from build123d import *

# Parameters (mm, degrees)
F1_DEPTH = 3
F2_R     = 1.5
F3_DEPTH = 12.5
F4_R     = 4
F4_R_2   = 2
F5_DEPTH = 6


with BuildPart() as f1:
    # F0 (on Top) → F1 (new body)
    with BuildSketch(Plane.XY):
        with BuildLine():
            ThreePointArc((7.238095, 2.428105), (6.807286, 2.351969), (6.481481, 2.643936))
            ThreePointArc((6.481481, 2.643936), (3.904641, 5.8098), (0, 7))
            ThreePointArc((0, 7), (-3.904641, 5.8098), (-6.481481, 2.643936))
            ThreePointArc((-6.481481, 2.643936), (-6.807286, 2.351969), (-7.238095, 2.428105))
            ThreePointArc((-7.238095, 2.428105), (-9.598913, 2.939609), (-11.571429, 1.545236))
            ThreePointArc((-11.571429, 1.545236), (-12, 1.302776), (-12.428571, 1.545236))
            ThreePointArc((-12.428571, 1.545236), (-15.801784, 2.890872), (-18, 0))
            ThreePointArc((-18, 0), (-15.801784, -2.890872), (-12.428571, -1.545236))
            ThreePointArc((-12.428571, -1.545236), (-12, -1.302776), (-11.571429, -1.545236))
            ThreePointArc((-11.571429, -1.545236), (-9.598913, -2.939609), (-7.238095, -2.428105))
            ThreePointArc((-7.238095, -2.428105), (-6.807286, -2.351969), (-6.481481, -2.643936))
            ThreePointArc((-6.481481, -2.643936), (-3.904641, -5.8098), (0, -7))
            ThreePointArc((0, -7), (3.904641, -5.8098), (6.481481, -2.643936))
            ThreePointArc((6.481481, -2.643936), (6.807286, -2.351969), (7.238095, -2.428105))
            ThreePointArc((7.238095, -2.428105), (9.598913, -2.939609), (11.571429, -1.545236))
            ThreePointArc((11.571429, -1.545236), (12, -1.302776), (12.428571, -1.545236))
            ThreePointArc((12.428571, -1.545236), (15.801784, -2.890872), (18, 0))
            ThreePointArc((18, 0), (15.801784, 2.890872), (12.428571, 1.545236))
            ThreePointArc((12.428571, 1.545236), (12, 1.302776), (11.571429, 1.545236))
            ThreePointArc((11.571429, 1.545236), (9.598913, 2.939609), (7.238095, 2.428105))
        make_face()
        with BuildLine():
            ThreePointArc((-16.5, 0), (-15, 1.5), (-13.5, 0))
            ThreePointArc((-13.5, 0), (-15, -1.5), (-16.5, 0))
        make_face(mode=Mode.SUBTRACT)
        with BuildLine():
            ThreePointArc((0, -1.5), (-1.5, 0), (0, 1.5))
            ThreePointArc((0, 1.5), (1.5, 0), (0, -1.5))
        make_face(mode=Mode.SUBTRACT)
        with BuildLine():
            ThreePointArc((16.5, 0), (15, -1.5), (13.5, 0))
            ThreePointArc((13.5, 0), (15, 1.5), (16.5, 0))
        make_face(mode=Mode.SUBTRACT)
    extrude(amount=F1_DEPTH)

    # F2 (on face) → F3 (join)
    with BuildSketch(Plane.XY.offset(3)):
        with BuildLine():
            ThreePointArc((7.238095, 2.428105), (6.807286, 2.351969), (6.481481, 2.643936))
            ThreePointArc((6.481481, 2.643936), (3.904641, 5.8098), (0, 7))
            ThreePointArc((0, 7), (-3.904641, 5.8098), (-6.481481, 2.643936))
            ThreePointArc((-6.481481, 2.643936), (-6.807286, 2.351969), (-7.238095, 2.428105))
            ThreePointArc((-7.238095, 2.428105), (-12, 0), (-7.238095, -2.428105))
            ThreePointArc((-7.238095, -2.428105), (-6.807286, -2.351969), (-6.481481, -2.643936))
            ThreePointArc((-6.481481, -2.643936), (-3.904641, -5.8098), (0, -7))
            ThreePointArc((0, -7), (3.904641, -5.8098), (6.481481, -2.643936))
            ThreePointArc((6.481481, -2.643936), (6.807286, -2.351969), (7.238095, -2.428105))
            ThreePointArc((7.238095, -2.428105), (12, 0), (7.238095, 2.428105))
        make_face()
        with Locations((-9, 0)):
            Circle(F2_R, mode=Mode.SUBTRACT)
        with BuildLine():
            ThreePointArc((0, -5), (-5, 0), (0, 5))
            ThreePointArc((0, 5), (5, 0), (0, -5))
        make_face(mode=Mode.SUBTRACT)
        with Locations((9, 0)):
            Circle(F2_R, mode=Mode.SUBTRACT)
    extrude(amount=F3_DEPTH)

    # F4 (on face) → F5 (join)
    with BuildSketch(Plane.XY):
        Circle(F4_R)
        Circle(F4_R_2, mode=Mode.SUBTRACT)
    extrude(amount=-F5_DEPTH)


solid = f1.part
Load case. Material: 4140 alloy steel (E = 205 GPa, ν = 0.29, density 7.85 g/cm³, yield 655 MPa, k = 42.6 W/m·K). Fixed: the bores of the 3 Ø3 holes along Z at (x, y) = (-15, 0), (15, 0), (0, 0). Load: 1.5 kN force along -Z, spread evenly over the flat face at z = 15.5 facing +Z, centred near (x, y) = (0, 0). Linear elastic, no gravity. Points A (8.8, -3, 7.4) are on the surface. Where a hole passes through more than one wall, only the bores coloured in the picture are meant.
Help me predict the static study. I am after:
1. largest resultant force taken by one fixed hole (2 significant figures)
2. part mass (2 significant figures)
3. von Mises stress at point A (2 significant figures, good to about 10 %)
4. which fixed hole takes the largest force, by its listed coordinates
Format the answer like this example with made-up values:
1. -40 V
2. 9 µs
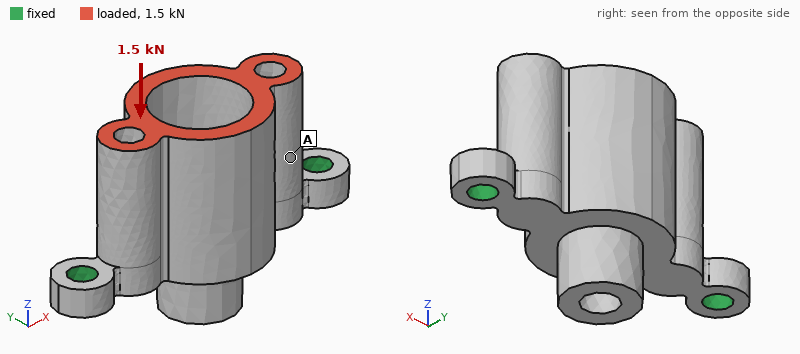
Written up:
1. 1.1 kN
2. 19 g
3. 13 MPa
4. (0, 0)
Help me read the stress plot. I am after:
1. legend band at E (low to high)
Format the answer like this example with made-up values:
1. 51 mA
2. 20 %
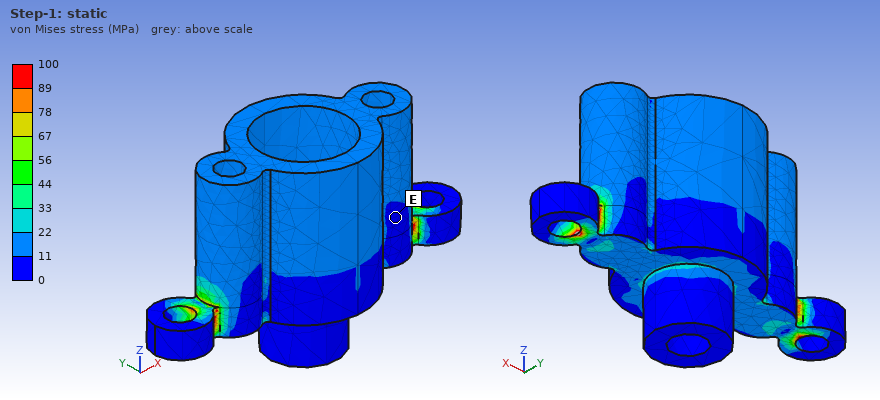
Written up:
1. 0 to 11 MPa
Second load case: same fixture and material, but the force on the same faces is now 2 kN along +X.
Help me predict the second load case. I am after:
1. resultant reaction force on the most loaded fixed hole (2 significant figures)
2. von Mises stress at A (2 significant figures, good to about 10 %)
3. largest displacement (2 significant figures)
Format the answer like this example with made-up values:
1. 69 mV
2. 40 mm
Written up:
1. 1.1 kN
2. 51 MPa
3. 18 µm
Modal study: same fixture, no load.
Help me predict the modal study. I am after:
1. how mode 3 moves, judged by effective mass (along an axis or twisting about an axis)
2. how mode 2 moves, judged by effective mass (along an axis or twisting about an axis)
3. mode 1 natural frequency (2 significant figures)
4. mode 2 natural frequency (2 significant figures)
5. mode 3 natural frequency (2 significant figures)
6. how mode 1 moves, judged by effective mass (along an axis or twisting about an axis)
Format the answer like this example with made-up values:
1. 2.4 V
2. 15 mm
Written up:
1. twisting about Z
2. along X
3. 11 kHz
4. 26 kHz
5. 27 kHz
6. along Y
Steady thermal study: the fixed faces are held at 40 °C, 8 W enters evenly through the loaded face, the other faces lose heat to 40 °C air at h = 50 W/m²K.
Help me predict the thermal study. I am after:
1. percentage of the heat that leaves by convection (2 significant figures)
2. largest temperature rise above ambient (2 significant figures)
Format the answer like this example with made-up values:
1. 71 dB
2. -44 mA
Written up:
1. 18 %
2. 27 K
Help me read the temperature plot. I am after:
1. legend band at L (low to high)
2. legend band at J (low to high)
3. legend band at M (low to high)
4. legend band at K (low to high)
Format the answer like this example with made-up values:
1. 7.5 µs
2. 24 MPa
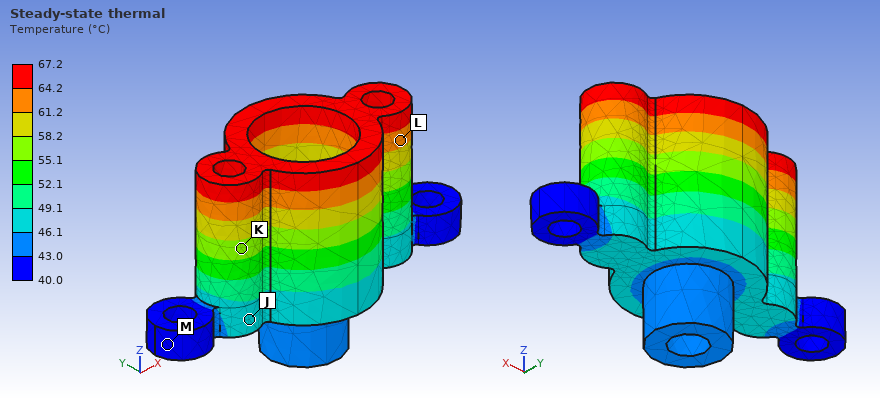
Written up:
1. 61.2 to 64.2 °C
2. 46.1 to 49.1 °C
3. 40.0 to 43.0 °C
4. 55.1 to 58.2 °C
